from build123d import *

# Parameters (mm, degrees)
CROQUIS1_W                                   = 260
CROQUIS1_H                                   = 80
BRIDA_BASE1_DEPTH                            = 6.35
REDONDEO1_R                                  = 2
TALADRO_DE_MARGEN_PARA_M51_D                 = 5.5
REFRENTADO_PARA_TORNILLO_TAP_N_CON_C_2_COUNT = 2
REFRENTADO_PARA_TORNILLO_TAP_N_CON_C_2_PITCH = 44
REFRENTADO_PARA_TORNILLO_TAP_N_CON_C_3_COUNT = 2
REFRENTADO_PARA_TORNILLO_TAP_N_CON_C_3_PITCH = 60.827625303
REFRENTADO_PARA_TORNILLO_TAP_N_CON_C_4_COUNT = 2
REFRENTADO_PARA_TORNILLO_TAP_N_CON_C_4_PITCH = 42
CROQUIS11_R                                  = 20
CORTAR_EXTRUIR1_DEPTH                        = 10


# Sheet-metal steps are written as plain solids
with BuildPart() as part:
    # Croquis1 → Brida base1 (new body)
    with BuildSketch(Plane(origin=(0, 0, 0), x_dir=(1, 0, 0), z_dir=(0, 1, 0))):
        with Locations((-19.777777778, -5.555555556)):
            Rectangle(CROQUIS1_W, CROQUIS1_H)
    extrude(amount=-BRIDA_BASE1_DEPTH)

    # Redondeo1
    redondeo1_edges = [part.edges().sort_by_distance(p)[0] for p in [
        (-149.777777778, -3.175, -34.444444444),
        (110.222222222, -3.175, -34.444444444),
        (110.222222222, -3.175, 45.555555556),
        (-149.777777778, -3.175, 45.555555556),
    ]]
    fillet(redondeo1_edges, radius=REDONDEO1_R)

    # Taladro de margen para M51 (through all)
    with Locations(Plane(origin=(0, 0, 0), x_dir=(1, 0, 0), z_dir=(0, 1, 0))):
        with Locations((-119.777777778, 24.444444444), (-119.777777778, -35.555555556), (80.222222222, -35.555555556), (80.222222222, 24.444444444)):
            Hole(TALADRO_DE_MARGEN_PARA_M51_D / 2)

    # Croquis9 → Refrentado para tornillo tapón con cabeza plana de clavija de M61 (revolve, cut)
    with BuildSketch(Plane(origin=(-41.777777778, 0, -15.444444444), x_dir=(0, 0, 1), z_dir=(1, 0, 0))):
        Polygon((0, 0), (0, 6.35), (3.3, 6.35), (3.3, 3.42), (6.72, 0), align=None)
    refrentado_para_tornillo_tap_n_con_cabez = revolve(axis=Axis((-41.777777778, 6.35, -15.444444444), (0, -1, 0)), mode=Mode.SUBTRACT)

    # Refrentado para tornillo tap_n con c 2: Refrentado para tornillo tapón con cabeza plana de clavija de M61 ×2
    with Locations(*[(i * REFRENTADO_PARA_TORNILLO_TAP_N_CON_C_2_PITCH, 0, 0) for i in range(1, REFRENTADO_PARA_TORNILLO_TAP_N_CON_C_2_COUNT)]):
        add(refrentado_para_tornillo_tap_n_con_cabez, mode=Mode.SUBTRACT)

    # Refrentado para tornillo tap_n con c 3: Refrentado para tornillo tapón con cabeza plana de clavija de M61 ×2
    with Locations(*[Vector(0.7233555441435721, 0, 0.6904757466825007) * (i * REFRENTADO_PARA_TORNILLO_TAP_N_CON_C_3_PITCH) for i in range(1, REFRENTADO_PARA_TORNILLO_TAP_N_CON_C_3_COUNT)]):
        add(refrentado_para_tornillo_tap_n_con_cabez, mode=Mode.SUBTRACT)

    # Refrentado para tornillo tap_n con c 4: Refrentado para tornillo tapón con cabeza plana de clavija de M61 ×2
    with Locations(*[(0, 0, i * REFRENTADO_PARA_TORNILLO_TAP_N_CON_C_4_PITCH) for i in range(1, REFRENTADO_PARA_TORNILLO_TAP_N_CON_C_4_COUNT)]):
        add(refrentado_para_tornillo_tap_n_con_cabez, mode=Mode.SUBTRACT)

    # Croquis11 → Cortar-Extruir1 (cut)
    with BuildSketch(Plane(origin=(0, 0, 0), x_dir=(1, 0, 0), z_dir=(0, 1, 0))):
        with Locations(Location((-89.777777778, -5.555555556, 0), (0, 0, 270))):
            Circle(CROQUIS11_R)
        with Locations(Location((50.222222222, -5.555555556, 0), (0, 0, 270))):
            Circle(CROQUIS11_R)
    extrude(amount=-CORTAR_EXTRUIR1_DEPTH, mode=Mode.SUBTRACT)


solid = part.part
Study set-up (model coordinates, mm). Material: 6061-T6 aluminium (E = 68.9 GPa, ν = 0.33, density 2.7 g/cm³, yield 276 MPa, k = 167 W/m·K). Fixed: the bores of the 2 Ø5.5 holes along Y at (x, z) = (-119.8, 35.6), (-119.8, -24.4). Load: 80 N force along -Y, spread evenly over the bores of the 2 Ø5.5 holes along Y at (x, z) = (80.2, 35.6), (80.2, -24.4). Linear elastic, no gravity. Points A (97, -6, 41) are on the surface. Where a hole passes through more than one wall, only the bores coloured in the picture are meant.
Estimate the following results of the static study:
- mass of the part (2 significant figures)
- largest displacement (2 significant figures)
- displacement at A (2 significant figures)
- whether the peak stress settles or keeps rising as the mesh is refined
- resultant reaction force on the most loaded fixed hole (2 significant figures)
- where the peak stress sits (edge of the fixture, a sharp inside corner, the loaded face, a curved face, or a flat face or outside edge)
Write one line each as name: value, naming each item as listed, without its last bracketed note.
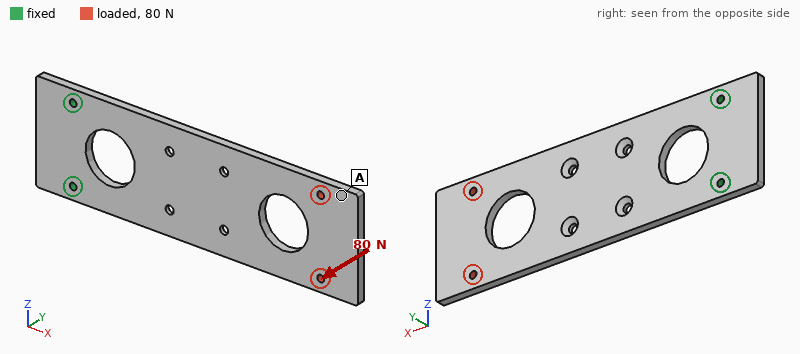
mass of the part: 310 g
largest displacement: 3.2 mm
displacement at A: 3.0 mm
whether the peak stress settles or keeps rising as the mesh is refined: keeps rising
resultant reaction force on the most loaded fixed hole: 40 N
where the peak stress sits: edge of the fixture
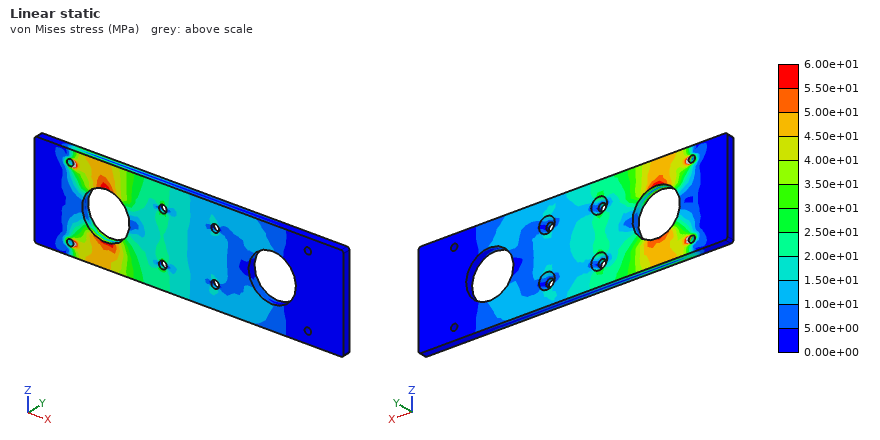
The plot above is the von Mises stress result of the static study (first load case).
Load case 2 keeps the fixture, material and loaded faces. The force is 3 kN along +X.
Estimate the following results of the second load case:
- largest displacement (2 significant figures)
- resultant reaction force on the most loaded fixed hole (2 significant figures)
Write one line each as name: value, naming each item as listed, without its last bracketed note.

largest displacement: 35 µm
resultant reaction force on the most loaded fixed hole: 1.5 kN
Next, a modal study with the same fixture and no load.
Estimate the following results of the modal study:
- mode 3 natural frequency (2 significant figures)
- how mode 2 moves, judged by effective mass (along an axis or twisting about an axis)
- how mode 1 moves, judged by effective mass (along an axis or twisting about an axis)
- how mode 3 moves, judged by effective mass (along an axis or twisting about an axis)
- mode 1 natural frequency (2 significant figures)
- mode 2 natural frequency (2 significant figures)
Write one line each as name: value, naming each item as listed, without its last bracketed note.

mode 3 natural frequency: 550 Hz
how mode 2 moves, judged by effective mass: twisting about X
how mode 1 moves, judged by effective mass: along Y
how mode 3 moves, judged by effective mass: along Y
mode 1 natural frequency: 86 Hz
mode 2 natural frequency: 520 Hz
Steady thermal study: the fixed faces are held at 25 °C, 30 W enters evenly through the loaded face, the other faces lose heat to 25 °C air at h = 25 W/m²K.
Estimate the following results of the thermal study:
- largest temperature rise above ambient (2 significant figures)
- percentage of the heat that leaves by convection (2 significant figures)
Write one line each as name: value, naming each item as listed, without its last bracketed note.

largest temperature rise above ambient: 49 K
percentage of the heat that leaves by convection: 70 %
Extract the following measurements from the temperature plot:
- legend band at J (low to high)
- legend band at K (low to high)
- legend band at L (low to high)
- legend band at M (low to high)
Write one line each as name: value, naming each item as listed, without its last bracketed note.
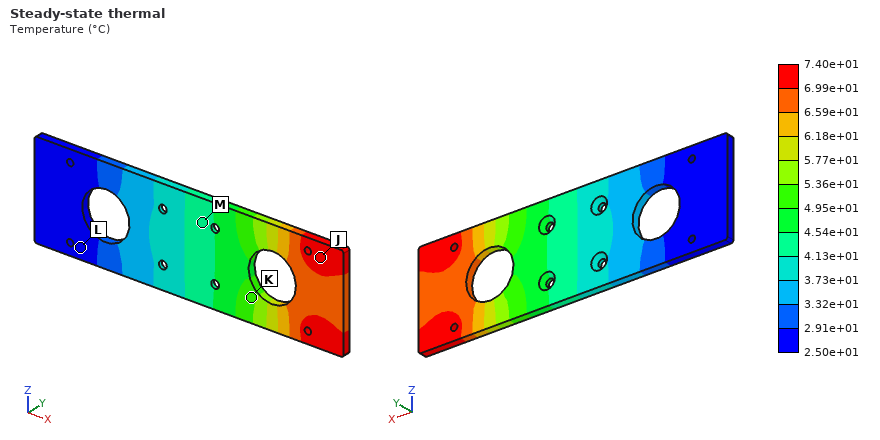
legend band at J: 6.99e+01 to 7.40e+01 °C
legend band at K: 4.95e+01 to 5.36e+01 °C
legend band at L: 2.50e+01 to 2.91e+01 °C
legend band at M: 4.13e+01 to 4.54e+01 °C
